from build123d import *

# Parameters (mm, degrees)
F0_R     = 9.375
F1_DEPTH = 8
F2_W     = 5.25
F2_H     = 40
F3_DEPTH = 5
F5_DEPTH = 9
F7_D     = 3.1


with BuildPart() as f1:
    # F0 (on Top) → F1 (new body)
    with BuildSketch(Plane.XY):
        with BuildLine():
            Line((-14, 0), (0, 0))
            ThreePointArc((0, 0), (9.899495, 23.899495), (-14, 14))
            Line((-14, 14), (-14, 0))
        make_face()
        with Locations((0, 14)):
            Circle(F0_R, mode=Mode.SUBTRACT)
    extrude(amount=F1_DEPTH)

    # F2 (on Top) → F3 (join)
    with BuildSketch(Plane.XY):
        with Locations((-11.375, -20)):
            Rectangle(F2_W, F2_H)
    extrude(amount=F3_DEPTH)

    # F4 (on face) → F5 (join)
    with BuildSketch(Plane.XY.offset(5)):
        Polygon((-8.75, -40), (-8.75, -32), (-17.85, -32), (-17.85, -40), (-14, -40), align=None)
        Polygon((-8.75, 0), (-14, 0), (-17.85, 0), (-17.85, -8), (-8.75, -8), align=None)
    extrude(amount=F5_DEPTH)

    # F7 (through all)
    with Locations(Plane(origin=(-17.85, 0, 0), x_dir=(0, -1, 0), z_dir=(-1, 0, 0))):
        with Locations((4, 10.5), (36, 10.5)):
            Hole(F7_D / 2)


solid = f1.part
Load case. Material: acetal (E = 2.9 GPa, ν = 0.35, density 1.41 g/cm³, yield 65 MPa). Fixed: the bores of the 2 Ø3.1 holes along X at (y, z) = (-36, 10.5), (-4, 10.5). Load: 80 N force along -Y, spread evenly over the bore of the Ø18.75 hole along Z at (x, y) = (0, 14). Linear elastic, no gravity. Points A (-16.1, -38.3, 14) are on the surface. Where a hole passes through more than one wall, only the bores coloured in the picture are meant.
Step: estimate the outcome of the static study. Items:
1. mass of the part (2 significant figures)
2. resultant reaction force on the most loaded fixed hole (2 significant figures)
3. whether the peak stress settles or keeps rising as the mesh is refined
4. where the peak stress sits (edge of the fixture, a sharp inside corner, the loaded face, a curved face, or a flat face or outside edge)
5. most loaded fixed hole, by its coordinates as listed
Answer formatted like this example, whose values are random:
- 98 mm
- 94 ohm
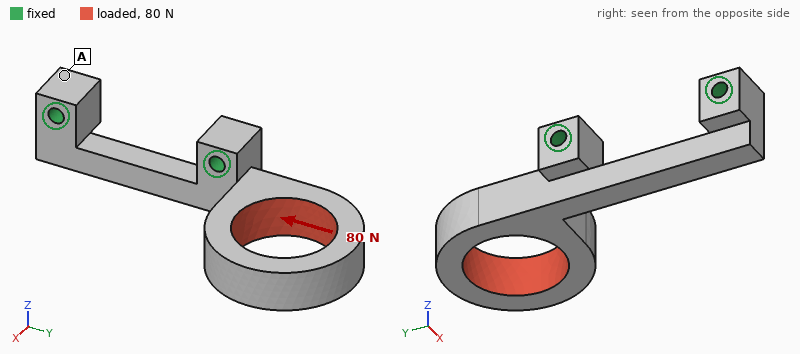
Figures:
- 7.4 g
- 55 N
- keeps rising
- a sharp inside corner
- (-4, 10.5)
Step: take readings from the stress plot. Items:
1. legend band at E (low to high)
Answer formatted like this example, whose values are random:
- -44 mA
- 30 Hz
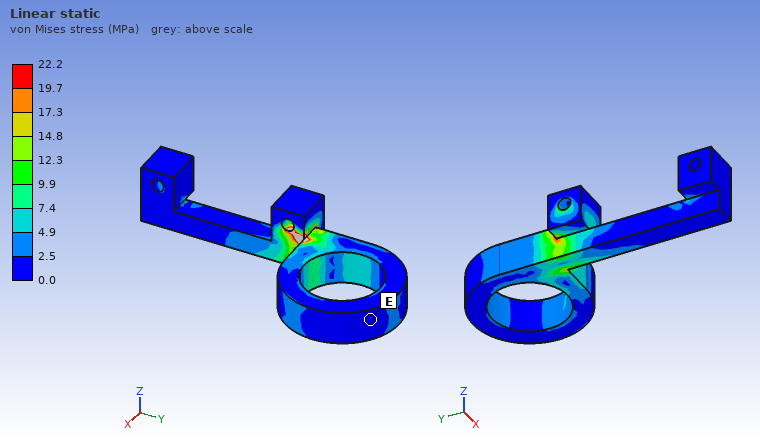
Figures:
- 0.0 to 2.5 MPa
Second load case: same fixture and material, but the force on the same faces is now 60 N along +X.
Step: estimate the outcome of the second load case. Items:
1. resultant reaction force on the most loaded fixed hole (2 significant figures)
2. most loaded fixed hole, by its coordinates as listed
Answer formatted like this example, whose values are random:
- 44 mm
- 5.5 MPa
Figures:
- 66 N
- (-4, 10.5)
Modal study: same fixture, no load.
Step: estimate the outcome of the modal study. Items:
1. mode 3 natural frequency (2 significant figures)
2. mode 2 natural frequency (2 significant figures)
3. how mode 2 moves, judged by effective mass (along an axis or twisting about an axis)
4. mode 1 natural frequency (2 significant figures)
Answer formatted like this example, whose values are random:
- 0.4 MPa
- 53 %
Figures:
- 1700 Hz
- 820 Hz
- along Z
- 700 Hz
